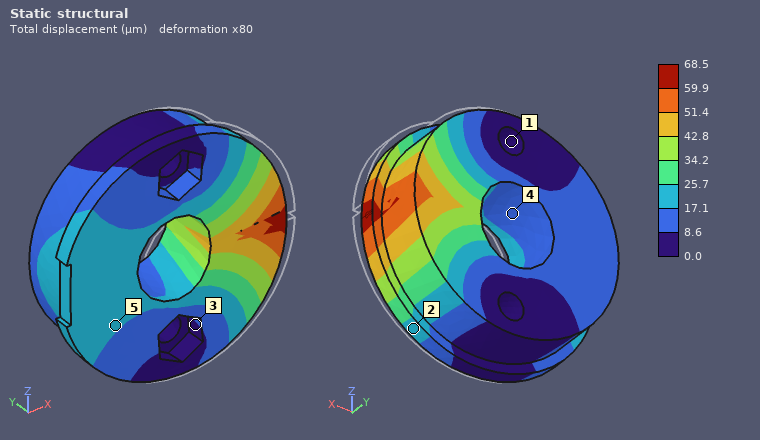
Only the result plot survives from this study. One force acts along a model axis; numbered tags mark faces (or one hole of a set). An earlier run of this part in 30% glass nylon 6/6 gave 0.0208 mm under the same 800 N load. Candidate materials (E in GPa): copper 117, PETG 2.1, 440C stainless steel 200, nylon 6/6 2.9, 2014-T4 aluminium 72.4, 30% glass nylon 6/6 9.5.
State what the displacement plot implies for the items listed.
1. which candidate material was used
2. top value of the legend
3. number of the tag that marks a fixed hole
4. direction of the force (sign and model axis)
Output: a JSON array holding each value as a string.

["nylon 6/6", "68.5 µm", "1", "-X"]
